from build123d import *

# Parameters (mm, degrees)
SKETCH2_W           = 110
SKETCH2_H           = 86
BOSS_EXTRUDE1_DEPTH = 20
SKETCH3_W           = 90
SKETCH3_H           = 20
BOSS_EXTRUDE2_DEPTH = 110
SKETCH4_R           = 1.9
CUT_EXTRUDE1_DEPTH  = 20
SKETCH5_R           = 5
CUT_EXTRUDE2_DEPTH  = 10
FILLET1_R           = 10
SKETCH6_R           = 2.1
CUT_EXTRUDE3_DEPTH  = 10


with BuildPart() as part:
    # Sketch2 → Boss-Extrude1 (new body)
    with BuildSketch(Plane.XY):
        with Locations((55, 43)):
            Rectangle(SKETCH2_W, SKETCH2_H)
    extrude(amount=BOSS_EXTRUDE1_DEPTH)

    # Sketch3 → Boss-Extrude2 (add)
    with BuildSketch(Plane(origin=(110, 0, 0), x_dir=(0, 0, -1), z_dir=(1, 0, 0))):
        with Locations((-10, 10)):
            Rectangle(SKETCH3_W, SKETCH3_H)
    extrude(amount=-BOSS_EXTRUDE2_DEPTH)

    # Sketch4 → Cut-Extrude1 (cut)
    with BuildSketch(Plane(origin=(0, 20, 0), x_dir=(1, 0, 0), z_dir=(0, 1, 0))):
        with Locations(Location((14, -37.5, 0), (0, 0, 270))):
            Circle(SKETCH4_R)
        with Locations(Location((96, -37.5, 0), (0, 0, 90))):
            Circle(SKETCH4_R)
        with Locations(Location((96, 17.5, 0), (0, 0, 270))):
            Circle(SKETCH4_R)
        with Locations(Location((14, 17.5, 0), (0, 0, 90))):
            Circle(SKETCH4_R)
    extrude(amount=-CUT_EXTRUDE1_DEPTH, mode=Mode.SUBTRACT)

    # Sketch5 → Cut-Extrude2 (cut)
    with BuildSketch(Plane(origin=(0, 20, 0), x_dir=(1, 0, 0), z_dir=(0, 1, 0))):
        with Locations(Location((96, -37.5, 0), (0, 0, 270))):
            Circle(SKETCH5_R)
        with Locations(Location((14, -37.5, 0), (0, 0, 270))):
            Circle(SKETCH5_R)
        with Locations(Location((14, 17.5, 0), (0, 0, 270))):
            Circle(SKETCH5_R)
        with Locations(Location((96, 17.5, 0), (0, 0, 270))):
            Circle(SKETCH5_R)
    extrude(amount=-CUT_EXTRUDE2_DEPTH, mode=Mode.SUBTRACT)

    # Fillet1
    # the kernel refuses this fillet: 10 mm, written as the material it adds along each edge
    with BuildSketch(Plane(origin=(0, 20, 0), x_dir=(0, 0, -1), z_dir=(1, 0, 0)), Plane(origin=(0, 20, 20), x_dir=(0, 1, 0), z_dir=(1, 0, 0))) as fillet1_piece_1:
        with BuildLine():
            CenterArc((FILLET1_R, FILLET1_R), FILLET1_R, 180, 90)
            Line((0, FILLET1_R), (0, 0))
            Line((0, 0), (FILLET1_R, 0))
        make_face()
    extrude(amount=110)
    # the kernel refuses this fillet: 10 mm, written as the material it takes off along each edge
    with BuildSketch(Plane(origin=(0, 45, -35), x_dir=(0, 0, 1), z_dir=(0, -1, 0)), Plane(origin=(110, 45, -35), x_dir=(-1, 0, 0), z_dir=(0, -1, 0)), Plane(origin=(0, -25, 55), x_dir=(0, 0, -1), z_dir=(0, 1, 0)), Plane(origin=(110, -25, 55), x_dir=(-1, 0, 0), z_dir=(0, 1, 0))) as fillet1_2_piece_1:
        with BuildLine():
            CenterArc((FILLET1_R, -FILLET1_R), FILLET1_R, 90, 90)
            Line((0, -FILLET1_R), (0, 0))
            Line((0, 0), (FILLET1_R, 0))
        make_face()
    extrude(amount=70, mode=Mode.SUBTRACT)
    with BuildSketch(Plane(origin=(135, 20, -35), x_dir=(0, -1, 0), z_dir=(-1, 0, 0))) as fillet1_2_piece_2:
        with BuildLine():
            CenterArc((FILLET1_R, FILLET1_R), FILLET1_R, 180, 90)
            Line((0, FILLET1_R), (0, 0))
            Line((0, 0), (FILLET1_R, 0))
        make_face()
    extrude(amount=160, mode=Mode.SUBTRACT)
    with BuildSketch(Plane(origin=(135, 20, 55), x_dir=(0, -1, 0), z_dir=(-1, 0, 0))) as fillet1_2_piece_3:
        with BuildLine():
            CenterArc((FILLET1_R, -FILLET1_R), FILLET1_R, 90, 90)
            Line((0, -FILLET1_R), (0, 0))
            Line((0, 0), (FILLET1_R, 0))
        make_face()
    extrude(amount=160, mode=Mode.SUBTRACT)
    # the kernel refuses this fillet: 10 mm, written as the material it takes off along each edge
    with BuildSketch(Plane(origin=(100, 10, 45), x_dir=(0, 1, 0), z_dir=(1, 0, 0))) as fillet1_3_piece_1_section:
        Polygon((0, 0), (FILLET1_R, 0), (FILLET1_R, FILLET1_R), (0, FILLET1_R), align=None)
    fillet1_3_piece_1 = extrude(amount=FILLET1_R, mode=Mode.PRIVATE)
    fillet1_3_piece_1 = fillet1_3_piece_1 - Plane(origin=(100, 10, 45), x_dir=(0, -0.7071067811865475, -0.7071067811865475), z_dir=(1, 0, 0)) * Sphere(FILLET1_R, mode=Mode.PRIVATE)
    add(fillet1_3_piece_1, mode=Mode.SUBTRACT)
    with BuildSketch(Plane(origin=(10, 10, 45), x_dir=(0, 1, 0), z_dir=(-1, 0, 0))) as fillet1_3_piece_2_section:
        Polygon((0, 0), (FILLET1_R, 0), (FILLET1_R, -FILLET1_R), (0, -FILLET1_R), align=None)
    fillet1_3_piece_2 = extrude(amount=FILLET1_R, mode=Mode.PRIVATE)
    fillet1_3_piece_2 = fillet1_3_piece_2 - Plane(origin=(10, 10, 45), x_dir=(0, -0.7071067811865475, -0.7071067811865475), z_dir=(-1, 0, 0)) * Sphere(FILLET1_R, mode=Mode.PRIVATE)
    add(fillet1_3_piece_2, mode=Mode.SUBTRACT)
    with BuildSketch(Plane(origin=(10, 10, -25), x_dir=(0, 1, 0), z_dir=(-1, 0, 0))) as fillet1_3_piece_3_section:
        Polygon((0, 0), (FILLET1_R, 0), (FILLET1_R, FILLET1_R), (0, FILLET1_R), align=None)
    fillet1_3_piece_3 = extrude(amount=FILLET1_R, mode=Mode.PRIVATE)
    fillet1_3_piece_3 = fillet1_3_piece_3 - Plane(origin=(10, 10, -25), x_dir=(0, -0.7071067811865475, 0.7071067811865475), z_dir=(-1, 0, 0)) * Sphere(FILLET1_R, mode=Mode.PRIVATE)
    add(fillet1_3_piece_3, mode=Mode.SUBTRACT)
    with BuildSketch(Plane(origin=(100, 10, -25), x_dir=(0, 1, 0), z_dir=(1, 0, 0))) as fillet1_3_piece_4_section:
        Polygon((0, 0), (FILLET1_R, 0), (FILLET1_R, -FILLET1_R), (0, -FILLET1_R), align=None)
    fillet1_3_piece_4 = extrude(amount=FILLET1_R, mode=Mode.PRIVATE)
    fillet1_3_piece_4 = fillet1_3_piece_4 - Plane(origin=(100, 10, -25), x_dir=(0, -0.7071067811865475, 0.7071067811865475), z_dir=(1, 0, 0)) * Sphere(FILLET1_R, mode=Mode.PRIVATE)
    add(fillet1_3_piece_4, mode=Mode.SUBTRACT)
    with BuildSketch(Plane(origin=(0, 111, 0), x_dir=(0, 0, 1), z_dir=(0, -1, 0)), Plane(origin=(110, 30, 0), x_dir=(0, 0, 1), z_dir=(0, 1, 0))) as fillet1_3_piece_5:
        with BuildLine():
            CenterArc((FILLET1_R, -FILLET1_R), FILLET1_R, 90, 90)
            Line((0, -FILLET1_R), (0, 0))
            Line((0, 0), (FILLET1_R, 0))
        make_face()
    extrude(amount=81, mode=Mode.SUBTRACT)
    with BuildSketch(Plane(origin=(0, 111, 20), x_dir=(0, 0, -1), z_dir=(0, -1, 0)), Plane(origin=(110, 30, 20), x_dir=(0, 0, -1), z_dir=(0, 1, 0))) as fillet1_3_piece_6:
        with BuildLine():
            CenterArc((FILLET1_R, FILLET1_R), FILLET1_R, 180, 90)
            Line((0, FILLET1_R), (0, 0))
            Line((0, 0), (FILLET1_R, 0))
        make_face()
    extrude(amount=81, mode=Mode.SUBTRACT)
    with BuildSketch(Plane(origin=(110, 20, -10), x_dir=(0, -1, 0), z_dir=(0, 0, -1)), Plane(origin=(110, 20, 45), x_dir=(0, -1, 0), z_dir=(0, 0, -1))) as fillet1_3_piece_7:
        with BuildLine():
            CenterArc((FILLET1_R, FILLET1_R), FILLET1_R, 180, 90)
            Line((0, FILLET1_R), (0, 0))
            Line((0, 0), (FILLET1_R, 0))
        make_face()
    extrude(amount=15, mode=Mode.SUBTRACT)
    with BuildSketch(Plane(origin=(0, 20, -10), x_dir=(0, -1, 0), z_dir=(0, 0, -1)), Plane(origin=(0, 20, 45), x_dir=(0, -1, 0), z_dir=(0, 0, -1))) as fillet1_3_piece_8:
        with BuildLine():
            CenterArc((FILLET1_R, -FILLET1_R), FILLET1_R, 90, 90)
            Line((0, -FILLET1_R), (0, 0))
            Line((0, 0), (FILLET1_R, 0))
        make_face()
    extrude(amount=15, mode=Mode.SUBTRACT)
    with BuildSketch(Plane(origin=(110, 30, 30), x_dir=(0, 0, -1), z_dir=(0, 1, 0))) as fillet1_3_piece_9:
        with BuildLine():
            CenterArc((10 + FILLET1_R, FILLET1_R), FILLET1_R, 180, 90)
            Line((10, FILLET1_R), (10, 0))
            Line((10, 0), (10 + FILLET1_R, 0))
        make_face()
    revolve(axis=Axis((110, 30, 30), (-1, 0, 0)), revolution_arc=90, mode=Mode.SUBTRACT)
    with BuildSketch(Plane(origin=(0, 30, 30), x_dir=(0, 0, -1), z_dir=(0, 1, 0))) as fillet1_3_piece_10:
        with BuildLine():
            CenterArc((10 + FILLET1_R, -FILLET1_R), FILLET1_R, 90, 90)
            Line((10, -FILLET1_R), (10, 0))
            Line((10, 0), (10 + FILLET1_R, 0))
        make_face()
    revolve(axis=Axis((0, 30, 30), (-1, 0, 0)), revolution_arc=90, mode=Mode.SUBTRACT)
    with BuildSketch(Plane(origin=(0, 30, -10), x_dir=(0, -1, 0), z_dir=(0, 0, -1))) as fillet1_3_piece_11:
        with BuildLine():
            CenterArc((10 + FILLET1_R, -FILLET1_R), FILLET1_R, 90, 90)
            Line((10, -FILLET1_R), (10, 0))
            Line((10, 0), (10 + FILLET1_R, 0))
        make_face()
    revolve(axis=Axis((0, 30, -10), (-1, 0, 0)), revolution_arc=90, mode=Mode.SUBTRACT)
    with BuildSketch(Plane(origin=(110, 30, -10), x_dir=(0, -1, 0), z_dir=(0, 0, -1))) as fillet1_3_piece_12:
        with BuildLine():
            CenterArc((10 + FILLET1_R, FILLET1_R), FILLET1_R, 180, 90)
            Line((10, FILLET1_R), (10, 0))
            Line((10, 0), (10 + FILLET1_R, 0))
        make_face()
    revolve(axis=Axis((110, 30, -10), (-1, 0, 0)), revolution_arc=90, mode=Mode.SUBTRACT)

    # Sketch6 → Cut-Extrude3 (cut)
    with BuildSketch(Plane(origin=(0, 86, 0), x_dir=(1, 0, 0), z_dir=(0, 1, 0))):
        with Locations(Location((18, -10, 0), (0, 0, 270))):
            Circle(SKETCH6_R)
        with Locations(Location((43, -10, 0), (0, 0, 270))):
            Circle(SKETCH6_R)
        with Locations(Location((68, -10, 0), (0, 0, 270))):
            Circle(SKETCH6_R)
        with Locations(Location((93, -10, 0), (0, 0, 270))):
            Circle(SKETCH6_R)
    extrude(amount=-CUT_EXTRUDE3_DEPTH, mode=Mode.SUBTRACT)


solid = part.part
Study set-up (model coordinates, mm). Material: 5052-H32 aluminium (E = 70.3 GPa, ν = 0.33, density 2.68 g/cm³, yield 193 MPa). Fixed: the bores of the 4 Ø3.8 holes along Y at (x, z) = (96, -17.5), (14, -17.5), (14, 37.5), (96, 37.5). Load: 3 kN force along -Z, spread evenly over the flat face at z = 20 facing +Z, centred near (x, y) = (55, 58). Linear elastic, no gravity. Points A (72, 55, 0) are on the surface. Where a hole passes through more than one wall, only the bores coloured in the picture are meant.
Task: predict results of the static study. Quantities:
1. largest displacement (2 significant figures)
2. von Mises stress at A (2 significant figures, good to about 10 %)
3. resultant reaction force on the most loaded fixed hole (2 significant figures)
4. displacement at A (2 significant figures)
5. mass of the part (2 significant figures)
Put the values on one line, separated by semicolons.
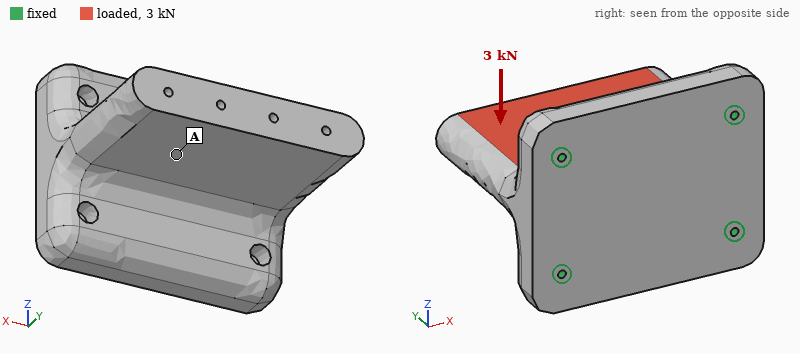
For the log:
39 µm; 3.8 MPa; 1.7 kN; 19 µm; 880 g
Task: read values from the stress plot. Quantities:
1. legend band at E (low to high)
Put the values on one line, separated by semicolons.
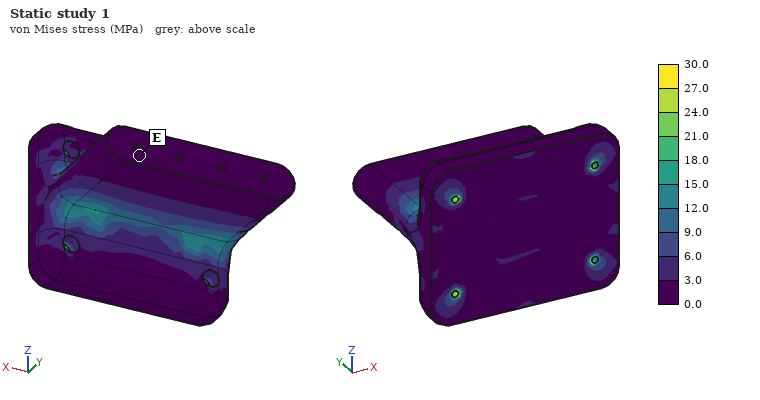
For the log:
0.0 to 3.0 MPa
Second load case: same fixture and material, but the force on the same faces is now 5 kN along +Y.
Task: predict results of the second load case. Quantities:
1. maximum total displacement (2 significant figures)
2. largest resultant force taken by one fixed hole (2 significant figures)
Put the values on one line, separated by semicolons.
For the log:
23 µm; 1.8 kN
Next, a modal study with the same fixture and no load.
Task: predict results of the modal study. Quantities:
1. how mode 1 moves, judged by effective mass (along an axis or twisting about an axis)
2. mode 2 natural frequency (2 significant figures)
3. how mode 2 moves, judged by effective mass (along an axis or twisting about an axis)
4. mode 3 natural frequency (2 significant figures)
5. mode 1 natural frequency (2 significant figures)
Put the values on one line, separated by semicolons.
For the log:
along Z; 5100 Hz; along X; 5400 Hz; 3100 Hz
